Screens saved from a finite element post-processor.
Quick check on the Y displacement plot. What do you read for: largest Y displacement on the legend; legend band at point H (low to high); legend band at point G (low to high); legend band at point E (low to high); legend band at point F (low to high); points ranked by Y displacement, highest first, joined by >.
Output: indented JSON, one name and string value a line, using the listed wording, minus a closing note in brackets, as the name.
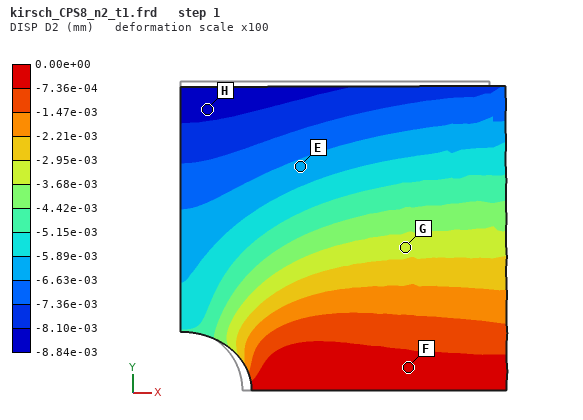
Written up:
{
  "largest Y displacement on the legend": "0.00e+00 mm",
  "legend band at point H": "-8.84e-03 to -8.10e-03 mm",
  "legend band at point G": "-3.68e-03 to -2.95e-03 mm",
  "legend band at point E": "-6.63e-03 to -5.89e-03 mm",
  "legend band at point F": "-7.36e-04 to 0.00e+00 mm",
  "points ranked by Y displacement, highest first, joined by >": "F > G > E > H"
}
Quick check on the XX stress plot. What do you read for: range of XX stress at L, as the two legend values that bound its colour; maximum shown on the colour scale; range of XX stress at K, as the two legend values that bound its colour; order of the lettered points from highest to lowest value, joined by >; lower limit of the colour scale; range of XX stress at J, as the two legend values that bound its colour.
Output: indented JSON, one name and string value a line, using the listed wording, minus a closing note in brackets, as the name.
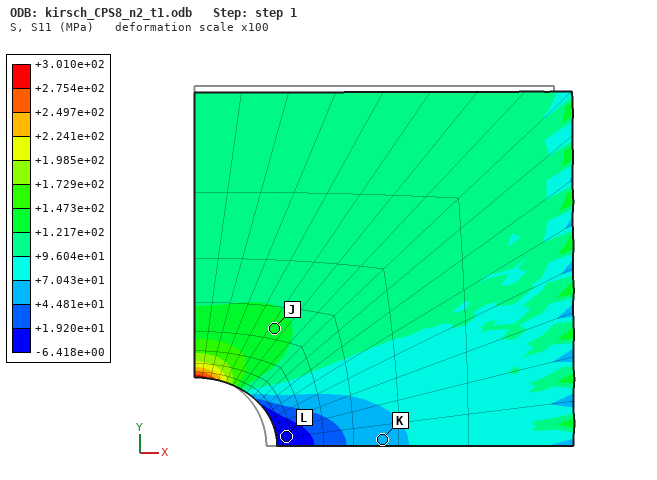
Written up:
{
  "range of XX stress at L, as the two legend values that bound its colour": "-6.418e+00 to +1.920e+01 MPa",
  "maximum shown on the colour scale": "+3.010e+02 MPa",
  "range of XX stress at K, as the two legend values that bound its colour": "+4.481e+01 to +7.043e+01 MPa",
  "order of the lettered points from highest to lowest value, joined by >": "J > K > L",
  "lower limit of the colour scale": "-6.418e+00 MPa",
  "range of XX stress at J, as the two legend values that bound its colour": "+1.217e+02 to +1.473e+02 MPa"
}
